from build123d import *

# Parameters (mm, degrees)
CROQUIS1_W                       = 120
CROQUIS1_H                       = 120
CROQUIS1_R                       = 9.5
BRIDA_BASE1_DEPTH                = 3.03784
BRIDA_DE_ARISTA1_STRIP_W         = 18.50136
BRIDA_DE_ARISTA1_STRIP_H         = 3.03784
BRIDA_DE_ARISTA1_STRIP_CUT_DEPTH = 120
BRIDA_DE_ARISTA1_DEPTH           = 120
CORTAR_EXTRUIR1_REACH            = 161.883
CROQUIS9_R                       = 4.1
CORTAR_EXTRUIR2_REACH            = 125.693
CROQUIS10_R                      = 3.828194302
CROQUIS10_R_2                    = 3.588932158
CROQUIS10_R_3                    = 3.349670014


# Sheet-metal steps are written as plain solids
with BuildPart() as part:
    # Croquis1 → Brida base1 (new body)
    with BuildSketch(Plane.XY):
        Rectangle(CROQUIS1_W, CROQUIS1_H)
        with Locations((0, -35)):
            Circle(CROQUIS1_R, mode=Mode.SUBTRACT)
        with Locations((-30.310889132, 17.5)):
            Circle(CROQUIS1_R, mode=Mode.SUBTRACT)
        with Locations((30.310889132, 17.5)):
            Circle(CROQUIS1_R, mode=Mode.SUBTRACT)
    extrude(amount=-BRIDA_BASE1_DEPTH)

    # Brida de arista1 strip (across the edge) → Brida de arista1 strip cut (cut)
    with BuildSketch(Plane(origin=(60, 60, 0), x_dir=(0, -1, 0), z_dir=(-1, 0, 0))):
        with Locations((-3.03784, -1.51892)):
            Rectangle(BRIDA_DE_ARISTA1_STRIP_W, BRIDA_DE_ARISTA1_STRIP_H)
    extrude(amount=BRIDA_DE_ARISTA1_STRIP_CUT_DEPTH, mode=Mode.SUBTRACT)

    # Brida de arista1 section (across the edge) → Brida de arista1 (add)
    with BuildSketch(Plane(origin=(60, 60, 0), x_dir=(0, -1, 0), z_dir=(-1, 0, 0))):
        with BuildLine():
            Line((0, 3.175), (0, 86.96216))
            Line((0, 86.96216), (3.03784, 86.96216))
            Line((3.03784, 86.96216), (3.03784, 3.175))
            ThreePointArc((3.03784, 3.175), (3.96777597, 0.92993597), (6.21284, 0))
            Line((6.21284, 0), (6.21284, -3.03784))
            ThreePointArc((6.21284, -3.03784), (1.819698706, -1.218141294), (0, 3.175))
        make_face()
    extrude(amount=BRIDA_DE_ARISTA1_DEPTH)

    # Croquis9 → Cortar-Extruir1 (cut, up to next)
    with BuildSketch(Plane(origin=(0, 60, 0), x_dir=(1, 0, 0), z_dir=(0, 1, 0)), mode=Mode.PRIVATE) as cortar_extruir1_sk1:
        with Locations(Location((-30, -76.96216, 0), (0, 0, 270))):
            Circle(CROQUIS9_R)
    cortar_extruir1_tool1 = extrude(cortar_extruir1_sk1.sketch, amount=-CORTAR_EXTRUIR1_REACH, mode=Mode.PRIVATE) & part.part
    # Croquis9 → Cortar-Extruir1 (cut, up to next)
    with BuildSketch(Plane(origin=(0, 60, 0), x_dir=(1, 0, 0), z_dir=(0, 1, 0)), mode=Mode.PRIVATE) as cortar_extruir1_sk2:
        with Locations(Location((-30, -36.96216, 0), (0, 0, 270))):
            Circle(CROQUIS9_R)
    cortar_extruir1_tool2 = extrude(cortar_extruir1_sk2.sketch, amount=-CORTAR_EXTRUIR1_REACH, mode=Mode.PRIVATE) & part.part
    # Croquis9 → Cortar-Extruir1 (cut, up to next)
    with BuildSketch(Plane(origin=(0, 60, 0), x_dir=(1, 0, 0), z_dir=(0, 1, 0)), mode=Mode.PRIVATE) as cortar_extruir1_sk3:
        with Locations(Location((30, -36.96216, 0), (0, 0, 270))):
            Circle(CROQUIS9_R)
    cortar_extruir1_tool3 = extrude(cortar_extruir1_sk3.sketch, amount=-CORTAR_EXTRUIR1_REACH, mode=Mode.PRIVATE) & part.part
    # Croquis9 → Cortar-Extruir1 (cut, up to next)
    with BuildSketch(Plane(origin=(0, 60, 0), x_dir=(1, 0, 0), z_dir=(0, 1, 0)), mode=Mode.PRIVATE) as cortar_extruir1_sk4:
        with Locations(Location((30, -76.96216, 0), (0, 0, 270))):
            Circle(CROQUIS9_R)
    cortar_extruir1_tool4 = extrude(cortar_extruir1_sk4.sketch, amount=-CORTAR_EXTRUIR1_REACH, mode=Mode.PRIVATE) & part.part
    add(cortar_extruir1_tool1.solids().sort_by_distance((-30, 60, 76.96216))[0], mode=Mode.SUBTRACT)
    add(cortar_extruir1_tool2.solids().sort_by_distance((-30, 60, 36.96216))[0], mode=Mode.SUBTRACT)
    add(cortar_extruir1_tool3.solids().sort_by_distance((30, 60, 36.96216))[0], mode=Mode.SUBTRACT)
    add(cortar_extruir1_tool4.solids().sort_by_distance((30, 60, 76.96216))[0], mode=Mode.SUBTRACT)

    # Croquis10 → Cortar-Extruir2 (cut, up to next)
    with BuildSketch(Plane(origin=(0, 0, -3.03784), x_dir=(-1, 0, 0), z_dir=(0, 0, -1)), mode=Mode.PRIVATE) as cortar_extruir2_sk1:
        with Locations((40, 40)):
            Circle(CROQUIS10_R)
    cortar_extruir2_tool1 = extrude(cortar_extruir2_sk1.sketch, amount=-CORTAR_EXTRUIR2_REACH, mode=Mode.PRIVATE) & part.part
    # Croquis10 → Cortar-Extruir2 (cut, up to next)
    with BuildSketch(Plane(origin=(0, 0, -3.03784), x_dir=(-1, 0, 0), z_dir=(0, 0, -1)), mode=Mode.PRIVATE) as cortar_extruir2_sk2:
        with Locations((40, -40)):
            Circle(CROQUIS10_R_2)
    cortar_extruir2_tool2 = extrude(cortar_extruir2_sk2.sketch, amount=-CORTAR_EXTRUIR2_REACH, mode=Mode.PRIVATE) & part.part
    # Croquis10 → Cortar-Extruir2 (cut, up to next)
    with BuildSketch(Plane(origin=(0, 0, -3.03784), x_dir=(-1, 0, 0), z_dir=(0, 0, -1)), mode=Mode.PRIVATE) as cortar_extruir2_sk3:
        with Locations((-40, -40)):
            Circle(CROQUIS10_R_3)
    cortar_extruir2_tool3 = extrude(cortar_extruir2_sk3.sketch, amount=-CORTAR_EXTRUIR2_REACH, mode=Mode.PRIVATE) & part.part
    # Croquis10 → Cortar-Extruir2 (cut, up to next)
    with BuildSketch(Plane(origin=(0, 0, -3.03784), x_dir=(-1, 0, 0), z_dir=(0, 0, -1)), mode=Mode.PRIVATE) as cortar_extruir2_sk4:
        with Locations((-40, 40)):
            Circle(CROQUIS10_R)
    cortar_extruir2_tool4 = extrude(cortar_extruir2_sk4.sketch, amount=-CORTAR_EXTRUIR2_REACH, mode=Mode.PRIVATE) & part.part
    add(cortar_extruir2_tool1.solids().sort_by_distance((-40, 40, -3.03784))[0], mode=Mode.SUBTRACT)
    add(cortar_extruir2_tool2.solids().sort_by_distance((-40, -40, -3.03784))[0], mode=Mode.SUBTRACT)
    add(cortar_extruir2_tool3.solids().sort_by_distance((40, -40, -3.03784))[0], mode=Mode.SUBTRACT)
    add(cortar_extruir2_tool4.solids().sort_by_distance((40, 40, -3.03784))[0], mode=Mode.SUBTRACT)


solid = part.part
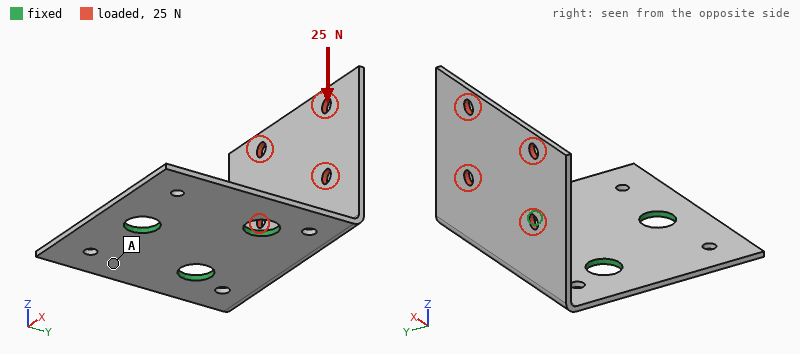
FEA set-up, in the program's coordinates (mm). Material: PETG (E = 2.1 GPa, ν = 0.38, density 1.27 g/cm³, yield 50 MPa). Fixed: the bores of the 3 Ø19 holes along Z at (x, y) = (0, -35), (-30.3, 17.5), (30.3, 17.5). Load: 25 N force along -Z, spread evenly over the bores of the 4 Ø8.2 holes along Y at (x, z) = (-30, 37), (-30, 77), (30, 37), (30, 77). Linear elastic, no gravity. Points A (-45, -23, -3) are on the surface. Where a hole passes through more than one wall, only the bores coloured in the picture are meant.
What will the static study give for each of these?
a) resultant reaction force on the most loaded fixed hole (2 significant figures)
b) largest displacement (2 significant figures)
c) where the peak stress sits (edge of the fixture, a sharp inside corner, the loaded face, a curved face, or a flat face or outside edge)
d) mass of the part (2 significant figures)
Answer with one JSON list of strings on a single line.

["13 N", "2.3 mm", "a flat face or outside edge", "90 g"]
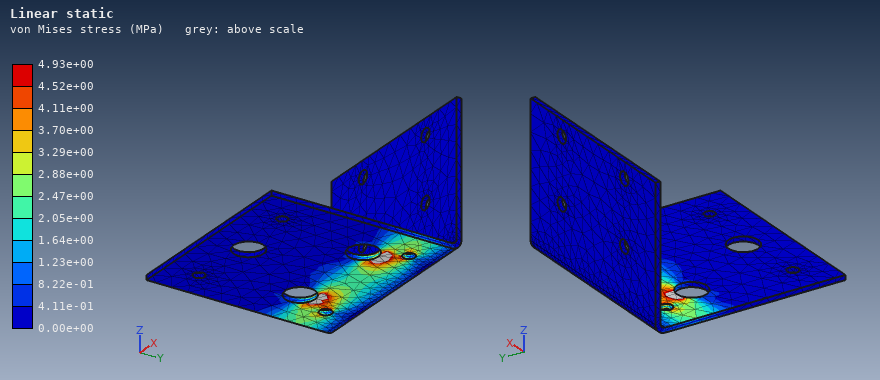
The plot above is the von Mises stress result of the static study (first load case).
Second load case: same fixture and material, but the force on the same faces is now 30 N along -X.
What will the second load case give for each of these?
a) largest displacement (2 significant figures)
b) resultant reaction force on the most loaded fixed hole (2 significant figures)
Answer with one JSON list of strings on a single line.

["2.2 mm", "32 N"]
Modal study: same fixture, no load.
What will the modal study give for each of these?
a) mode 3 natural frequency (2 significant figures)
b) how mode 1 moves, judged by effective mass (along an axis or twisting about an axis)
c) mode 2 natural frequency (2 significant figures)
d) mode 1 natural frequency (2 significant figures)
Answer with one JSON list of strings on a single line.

["170 Hz", "along Y", "110 Hz", "52 Hz"]
